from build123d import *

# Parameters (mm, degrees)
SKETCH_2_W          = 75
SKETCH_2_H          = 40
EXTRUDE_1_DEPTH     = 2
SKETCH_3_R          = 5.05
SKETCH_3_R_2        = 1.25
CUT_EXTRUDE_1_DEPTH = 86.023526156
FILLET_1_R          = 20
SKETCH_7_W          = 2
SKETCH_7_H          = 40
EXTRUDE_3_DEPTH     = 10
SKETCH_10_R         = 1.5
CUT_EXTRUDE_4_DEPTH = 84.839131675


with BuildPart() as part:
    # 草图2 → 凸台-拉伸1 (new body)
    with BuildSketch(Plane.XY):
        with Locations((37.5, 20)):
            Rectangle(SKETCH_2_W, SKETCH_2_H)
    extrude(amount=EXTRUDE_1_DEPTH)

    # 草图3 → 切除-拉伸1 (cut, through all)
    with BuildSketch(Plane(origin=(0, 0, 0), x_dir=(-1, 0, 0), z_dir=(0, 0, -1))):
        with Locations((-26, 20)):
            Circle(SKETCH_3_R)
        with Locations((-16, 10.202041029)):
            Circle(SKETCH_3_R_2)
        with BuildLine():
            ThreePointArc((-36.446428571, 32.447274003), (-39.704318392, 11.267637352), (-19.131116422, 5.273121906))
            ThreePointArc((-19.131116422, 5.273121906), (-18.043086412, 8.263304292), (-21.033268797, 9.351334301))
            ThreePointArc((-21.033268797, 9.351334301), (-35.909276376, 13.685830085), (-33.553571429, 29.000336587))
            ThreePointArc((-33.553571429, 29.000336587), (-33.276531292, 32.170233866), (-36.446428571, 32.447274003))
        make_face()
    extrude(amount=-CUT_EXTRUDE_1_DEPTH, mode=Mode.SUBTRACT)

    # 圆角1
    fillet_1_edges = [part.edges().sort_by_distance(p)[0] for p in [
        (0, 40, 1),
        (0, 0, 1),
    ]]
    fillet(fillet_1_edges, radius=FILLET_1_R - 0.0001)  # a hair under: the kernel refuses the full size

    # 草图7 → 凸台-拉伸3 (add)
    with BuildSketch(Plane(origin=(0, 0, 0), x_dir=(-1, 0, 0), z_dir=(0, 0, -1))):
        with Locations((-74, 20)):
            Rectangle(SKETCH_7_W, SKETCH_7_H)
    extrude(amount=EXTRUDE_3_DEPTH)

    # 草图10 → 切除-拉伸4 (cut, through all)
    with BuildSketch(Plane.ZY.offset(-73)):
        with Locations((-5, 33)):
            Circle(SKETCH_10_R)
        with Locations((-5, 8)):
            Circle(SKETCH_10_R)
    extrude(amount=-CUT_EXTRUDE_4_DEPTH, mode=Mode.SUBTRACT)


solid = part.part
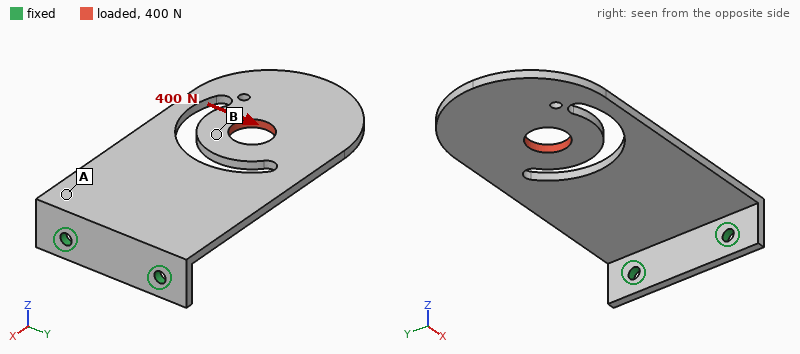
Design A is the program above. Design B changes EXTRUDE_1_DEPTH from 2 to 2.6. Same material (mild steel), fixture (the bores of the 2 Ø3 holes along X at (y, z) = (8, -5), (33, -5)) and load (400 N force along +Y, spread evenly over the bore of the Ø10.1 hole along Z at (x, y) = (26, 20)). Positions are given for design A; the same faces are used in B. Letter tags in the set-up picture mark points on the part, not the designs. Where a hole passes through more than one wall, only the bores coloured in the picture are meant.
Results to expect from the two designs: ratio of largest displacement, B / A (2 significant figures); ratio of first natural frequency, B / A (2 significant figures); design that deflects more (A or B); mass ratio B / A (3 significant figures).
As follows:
0.88
1.1
A
1.26
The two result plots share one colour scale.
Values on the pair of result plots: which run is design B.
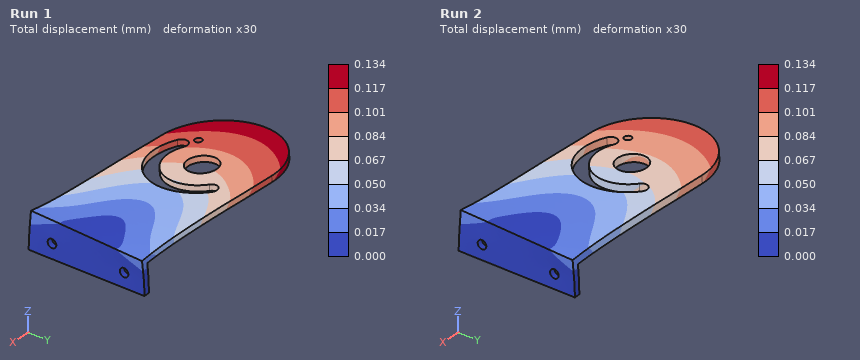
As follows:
Run 2
